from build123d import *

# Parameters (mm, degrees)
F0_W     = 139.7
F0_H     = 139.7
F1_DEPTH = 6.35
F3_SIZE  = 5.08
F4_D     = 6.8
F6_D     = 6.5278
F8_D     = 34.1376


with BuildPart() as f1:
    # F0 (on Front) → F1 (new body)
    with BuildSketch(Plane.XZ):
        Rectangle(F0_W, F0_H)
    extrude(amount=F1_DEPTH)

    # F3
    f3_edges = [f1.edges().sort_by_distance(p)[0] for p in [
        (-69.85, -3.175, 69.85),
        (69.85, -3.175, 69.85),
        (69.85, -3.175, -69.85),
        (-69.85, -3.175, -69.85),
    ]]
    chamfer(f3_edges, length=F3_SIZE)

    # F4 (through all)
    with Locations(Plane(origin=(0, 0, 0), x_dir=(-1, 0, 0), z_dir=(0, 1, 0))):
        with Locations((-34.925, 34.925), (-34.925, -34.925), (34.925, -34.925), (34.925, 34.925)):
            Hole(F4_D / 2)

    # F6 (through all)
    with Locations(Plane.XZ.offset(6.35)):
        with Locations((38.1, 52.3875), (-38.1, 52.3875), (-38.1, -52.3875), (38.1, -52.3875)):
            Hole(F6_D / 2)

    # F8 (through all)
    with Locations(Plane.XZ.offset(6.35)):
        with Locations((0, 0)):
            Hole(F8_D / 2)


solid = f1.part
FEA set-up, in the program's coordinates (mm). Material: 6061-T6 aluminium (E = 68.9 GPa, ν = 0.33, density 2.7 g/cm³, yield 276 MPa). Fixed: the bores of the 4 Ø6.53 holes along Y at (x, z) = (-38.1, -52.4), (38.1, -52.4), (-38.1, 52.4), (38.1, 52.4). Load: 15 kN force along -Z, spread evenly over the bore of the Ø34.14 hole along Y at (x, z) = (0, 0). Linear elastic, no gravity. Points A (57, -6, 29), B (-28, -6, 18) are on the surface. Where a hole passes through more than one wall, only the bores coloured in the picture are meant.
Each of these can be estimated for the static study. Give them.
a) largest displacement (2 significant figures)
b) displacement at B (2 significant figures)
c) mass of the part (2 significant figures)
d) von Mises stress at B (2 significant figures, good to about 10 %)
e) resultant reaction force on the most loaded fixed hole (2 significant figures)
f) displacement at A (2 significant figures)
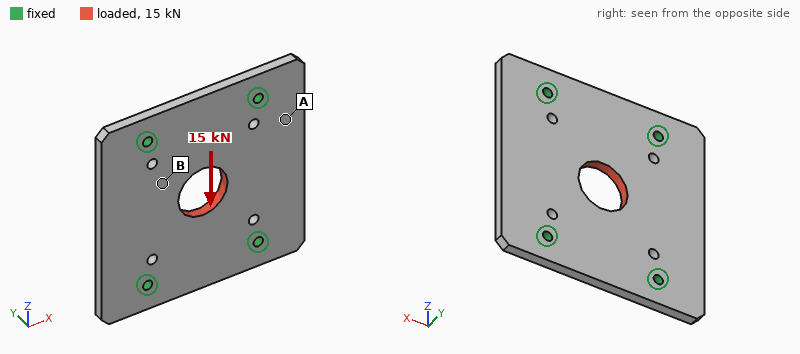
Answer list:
19 µm
11 µm
310 g
14 MPa
3.9 kN
5.0 µm
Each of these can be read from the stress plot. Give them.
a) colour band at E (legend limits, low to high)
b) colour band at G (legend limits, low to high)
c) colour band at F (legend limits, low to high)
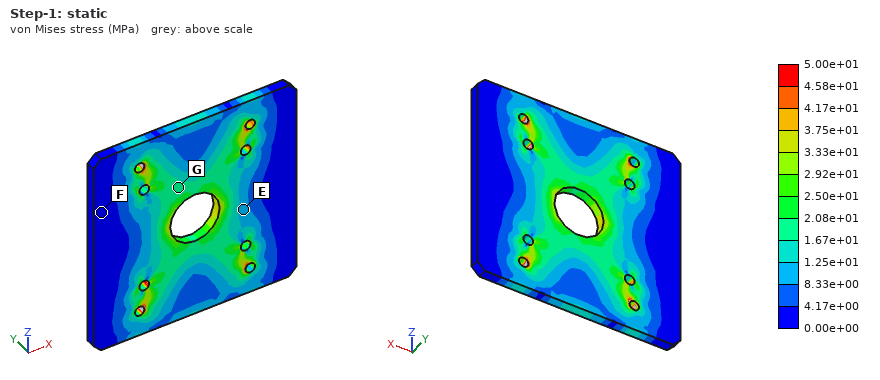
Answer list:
8.33e+00 to 1.25e+01 MPa
1.67e+01 to 2.08e+01 MPa
0.00e+00 to 4.17e+00 MPa
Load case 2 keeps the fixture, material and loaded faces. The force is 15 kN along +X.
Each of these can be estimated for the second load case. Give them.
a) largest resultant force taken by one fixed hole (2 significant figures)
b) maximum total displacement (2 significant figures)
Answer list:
3.9 kN
25 µm
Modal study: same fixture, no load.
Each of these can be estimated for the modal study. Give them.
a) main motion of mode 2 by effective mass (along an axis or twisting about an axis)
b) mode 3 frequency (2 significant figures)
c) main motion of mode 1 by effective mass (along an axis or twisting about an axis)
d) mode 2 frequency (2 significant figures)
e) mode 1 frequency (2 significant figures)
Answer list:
twisting about Z
3100 Hz
along Y
2500 Hz
2400 Hz
